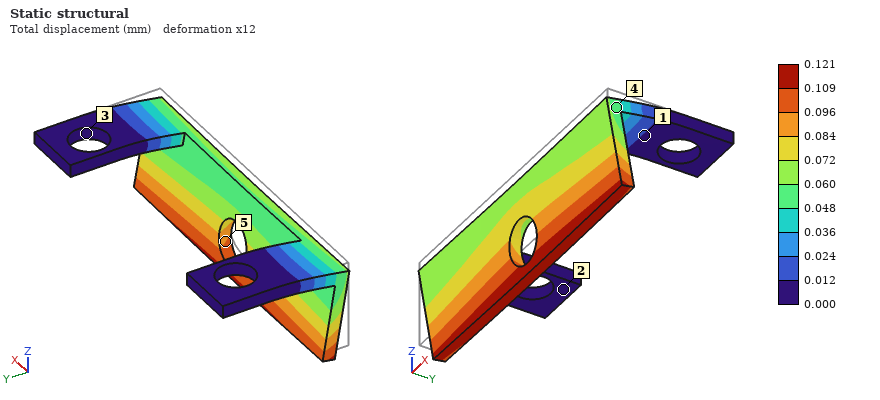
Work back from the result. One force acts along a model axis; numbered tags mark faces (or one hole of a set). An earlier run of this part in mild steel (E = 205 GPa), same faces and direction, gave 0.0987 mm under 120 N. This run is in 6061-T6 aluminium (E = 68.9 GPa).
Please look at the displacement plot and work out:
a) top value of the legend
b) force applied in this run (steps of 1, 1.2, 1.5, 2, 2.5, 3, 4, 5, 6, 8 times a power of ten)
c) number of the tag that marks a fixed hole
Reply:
0.121 mm
50 N
3
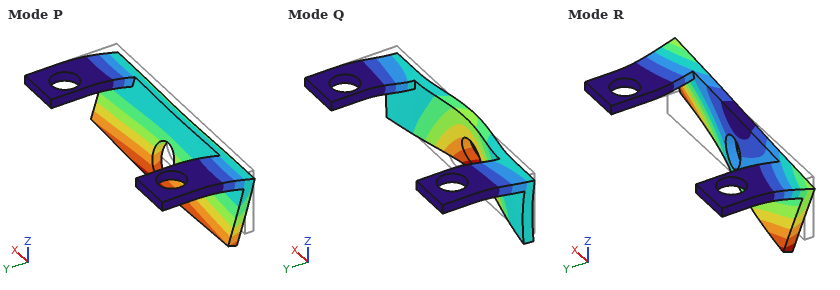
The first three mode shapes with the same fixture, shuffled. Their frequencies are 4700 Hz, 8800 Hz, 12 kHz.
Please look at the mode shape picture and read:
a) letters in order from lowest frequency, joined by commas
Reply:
P, R, Q
